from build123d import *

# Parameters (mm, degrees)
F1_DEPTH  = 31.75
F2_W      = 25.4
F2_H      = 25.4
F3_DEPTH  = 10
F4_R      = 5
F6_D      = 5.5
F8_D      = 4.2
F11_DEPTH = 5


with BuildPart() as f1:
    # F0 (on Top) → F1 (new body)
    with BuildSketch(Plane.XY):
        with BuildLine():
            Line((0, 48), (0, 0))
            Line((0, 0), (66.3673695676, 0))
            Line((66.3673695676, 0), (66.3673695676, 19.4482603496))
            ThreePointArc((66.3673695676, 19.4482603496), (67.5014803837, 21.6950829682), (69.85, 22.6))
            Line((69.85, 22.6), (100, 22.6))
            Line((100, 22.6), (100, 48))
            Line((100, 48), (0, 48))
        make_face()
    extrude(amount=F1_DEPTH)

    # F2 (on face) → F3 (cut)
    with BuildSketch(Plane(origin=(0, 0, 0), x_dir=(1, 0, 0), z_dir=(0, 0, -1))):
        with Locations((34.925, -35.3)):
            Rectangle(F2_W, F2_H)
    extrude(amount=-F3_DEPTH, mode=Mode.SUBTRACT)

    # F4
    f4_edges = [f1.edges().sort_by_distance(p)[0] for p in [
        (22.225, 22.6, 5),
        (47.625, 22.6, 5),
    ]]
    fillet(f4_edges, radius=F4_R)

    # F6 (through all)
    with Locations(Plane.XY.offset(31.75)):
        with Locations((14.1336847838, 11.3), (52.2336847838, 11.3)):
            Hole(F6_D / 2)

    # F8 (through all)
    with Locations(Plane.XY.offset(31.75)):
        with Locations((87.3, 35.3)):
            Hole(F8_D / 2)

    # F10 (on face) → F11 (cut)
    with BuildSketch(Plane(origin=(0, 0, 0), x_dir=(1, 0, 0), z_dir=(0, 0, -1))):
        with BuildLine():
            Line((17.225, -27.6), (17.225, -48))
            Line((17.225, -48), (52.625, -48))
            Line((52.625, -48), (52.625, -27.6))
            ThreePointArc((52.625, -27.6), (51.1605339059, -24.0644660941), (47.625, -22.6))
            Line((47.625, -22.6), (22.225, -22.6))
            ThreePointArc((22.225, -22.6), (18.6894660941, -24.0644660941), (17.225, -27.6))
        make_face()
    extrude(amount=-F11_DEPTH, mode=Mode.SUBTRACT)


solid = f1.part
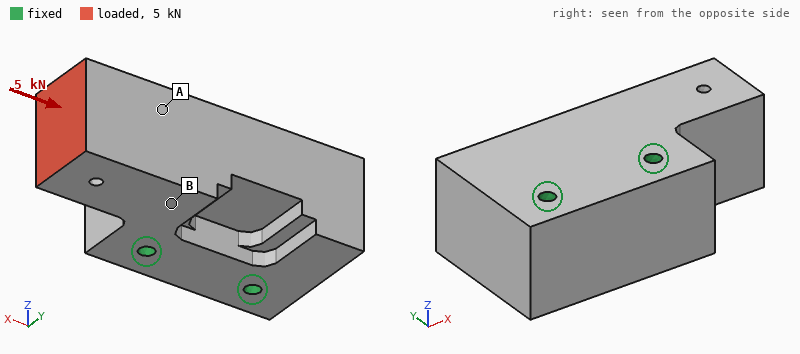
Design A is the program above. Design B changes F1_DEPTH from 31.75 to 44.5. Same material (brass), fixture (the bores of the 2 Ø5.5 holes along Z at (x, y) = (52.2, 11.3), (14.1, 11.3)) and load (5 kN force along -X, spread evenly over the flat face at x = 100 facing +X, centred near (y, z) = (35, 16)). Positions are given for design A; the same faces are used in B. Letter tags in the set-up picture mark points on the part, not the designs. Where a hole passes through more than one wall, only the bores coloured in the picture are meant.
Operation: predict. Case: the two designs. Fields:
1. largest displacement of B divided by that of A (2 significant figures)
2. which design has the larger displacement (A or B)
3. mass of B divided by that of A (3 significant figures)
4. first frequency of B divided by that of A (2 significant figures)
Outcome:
0.66
A
1.43
1.2
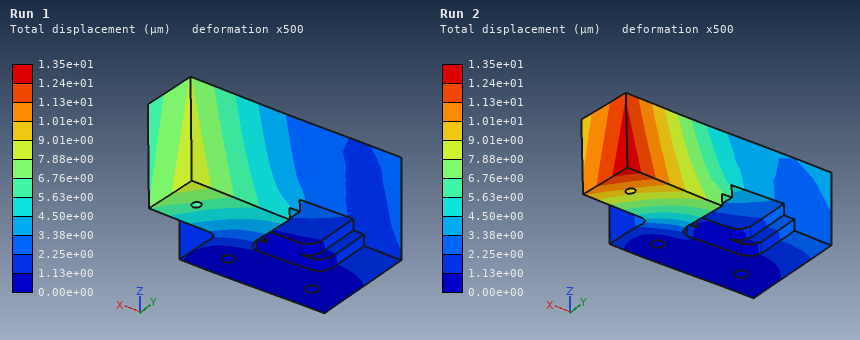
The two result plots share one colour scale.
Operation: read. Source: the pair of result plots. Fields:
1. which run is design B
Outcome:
Run 1
